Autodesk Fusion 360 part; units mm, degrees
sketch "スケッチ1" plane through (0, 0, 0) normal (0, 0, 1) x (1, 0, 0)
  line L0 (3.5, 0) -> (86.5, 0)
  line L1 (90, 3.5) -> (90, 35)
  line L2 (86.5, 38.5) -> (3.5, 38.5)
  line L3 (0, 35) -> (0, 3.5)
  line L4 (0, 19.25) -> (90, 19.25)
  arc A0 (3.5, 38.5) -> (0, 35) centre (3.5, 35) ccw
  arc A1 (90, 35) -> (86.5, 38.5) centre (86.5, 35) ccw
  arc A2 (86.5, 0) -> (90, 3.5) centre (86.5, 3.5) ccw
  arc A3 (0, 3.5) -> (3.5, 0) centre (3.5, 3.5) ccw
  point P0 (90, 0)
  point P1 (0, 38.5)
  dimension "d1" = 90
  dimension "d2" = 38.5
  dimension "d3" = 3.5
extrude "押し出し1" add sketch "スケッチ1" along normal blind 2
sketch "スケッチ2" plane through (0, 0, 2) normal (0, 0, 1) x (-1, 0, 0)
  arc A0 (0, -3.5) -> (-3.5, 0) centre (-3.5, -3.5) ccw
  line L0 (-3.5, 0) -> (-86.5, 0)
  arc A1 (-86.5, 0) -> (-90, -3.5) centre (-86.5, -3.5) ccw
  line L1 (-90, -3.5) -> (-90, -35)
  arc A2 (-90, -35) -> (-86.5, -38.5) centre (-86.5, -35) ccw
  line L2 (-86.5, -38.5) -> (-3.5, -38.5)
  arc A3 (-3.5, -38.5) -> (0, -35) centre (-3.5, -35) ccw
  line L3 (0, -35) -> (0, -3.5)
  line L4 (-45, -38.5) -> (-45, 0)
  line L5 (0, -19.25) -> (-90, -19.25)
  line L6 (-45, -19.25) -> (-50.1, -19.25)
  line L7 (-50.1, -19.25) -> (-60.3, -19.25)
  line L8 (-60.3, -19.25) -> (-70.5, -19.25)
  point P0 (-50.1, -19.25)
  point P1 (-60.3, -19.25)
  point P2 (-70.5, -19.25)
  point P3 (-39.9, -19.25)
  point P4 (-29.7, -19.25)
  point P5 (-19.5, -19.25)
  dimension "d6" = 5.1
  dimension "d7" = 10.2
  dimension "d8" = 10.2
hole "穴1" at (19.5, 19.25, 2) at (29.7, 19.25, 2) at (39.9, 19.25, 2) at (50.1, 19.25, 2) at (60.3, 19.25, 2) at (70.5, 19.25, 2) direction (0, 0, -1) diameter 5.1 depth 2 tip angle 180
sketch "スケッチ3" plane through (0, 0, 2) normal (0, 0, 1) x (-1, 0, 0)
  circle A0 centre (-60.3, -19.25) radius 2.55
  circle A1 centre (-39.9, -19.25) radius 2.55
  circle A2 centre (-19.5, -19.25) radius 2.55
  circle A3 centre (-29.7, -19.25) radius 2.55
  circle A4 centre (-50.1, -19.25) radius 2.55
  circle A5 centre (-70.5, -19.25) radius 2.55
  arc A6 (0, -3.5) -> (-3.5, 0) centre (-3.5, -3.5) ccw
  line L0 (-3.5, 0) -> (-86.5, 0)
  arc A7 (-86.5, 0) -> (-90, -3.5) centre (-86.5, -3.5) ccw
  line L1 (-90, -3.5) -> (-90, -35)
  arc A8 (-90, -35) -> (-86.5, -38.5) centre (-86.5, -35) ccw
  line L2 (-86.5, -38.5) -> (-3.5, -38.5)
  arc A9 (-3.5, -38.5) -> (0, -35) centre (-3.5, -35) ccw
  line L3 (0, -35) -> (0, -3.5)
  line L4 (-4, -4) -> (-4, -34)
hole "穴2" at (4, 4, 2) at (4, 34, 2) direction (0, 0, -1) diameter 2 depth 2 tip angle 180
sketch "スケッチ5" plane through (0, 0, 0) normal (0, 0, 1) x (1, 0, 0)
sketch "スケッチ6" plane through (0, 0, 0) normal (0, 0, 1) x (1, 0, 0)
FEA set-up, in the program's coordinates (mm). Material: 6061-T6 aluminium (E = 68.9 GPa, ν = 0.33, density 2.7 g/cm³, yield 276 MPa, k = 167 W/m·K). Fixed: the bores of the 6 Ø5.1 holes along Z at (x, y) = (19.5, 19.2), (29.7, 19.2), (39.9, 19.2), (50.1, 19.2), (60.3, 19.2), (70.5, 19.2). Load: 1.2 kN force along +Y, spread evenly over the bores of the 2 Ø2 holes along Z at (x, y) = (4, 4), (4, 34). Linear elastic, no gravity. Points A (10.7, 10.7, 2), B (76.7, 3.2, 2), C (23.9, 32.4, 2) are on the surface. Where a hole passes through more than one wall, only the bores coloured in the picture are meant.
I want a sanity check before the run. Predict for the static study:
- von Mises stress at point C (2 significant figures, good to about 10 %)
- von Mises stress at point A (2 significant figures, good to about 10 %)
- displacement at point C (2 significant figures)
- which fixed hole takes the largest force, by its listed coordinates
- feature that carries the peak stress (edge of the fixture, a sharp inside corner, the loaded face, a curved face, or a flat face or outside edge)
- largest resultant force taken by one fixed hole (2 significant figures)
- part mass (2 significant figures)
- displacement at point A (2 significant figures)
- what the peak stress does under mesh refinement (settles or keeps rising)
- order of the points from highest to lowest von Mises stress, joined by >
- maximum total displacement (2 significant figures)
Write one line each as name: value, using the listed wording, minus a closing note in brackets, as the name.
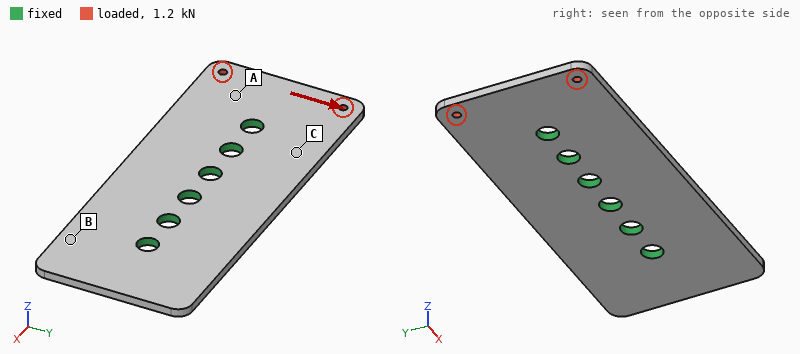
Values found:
von Mises stress at point C: 22 MPa
von Mises stress at point A: 35 MPa
displacement at point C: 6.0 µm
which fixed hole takes the largest force, by its listed coordinates: (19.5, 19.2)
feature that carries the peak stress: edge of the fixture
largest resultant force taken by one fixed hole: 1.6 kN
part mass: 18 g
displacement at point A: 14 µm
what the peak stress does under mesh refinement: keeps rising
order of the points from highest to lowest von Mises stress, joined by >: A > C > B
maximum total displacement: 32 µm
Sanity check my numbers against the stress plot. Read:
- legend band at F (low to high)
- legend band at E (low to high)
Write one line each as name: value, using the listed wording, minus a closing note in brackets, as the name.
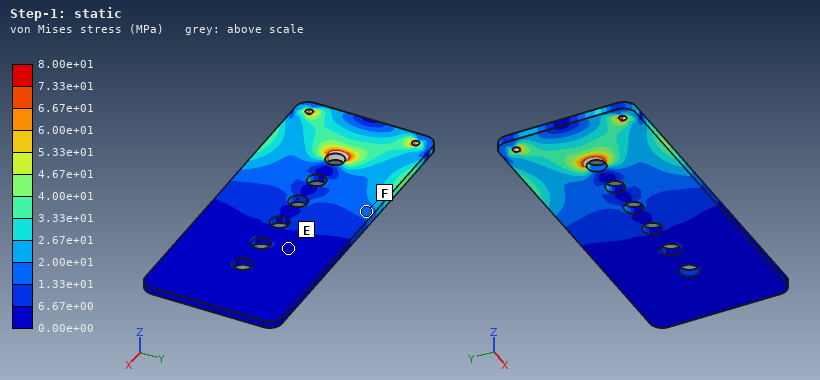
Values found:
legend band at F: 1.33e+01 to 2.00e+01 MPa
legend band at E: 0.00e+00 to 6.67e+00 MPa
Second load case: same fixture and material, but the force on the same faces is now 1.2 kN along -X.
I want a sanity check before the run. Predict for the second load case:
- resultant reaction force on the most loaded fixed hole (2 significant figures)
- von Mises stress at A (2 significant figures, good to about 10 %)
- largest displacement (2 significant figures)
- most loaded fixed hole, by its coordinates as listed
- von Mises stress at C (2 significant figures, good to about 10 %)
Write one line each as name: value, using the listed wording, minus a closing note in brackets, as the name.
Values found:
resultant reaction force on the most loaded fixed hole: 600 N
von Mises stress at A: 20 MPa
largest displacement: 12 µm
most loaded fixed hole, by its coordinates as listed: (19.5, 19.2)
von Mises stress at C: 13 MPa
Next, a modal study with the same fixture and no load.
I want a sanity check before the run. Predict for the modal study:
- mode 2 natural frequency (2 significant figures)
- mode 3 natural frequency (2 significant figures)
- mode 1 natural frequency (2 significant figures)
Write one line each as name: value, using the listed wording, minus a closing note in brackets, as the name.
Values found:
mode 2 natural frequency: 3900 Hz
mode 3 natural frequency: 3900 Hz
mode 1 natural frequency: 3900 Hz
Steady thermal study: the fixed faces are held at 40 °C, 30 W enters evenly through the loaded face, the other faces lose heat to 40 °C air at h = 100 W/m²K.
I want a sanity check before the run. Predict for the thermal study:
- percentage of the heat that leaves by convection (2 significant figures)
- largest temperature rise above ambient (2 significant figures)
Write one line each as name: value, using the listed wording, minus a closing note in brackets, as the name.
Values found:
percentage of the heat that leaves by convection: 18 %
largest temperature rise above ambient: 59 K
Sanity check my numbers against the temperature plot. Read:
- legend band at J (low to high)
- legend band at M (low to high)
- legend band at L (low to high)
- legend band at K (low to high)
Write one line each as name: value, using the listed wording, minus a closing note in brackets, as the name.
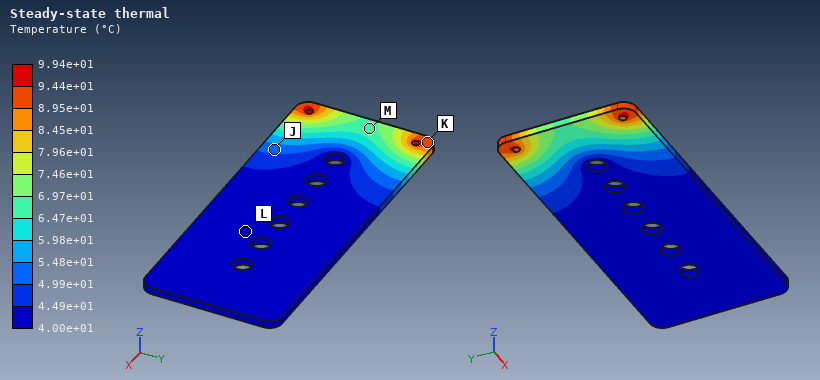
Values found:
legend band at J: 4.99e+01 to 5.48e+01 °C
legend band at M: 6.47e+01 to 6.97e+01 °C
legend band at L: 4.00e+01 to 4.49e+01 °C
legend band at K: 8.95e+01 to 9.44e+01 °C
